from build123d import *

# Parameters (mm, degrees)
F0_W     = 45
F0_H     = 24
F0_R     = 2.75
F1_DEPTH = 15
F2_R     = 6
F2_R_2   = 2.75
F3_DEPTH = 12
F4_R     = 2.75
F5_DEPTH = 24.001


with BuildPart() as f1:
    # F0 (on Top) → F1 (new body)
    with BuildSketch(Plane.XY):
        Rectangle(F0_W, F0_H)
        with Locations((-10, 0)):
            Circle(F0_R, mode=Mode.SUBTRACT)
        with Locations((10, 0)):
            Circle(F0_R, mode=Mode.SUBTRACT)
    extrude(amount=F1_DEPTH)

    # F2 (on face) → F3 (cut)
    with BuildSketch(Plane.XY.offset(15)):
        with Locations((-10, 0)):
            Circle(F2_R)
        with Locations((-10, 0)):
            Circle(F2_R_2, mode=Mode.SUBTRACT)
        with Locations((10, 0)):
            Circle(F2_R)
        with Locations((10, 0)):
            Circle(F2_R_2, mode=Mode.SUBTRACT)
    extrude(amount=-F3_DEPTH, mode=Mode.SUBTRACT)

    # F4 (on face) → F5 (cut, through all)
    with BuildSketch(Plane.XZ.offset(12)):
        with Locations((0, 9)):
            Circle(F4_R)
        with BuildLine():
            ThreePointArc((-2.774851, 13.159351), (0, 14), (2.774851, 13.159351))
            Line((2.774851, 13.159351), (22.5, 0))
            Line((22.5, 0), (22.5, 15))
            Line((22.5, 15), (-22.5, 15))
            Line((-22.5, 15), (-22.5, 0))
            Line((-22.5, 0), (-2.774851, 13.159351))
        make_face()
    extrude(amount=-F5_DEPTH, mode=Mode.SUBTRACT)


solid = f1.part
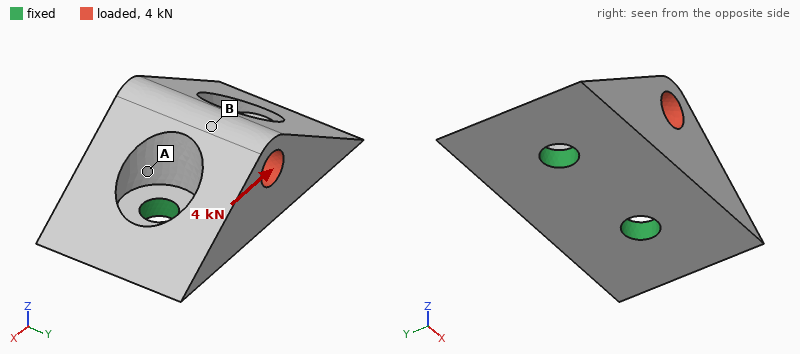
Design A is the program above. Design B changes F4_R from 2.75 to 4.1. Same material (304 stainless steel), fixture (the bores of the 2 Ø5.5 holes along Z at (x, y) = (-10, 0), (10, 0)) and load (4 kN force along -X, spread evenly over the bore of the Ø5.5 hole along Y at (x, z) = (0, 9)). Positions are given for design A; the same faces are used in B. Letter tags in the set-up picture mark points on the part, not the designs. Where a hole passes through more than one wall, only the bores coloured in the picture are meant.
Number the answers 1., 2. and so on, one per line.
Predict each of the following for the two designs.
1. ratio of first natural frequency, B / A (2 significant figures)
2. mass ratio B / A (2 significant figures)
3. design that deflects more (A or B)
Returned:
1. 1.1
2. 0.89
3. B
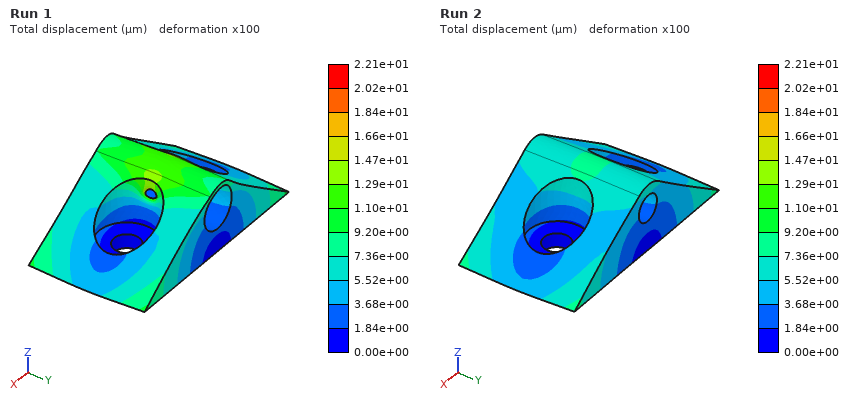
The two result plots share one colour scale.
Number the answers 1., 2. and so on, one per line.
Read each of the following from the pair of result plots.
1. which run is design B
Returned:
1. Run 1
